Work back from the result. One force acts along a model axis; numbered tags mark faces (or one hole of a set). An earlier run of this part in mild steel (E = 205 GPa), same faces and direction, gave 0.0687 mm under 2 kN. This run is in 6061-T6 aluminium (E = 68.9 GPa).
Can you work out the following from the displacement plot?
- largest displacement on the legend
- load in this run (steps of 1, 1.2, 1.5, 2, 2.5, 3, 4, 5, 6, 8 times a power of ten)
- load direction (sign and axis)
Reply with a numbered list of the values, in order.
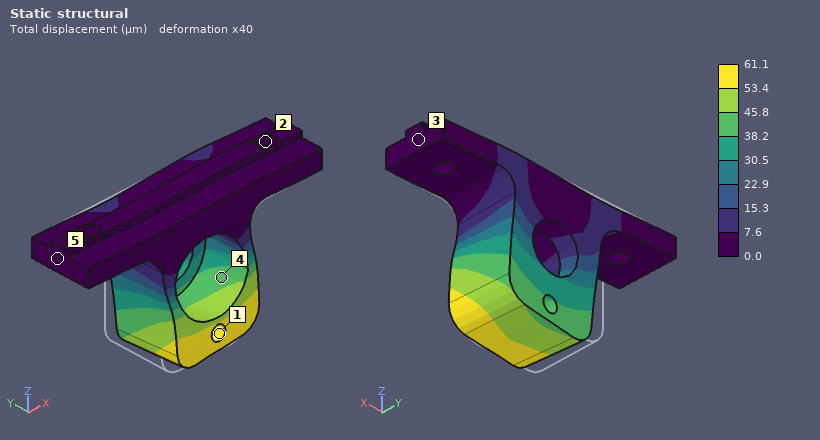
1. 61.1 µm
2. 600 N
3. +X
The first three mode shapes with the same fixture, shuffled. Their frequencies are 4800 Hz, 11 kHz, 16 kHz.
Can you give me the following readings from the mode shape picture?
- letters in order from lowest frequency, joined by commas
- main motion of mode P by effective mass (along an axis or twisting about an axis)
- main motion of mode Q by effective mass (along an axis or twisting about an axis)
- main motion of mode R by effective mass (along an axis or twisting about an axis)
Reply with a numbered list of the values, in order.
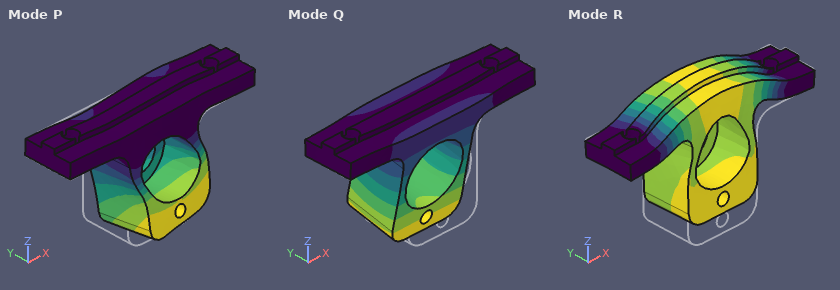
1. Q, P, R
2. along X
3. along Y
4. along Z
